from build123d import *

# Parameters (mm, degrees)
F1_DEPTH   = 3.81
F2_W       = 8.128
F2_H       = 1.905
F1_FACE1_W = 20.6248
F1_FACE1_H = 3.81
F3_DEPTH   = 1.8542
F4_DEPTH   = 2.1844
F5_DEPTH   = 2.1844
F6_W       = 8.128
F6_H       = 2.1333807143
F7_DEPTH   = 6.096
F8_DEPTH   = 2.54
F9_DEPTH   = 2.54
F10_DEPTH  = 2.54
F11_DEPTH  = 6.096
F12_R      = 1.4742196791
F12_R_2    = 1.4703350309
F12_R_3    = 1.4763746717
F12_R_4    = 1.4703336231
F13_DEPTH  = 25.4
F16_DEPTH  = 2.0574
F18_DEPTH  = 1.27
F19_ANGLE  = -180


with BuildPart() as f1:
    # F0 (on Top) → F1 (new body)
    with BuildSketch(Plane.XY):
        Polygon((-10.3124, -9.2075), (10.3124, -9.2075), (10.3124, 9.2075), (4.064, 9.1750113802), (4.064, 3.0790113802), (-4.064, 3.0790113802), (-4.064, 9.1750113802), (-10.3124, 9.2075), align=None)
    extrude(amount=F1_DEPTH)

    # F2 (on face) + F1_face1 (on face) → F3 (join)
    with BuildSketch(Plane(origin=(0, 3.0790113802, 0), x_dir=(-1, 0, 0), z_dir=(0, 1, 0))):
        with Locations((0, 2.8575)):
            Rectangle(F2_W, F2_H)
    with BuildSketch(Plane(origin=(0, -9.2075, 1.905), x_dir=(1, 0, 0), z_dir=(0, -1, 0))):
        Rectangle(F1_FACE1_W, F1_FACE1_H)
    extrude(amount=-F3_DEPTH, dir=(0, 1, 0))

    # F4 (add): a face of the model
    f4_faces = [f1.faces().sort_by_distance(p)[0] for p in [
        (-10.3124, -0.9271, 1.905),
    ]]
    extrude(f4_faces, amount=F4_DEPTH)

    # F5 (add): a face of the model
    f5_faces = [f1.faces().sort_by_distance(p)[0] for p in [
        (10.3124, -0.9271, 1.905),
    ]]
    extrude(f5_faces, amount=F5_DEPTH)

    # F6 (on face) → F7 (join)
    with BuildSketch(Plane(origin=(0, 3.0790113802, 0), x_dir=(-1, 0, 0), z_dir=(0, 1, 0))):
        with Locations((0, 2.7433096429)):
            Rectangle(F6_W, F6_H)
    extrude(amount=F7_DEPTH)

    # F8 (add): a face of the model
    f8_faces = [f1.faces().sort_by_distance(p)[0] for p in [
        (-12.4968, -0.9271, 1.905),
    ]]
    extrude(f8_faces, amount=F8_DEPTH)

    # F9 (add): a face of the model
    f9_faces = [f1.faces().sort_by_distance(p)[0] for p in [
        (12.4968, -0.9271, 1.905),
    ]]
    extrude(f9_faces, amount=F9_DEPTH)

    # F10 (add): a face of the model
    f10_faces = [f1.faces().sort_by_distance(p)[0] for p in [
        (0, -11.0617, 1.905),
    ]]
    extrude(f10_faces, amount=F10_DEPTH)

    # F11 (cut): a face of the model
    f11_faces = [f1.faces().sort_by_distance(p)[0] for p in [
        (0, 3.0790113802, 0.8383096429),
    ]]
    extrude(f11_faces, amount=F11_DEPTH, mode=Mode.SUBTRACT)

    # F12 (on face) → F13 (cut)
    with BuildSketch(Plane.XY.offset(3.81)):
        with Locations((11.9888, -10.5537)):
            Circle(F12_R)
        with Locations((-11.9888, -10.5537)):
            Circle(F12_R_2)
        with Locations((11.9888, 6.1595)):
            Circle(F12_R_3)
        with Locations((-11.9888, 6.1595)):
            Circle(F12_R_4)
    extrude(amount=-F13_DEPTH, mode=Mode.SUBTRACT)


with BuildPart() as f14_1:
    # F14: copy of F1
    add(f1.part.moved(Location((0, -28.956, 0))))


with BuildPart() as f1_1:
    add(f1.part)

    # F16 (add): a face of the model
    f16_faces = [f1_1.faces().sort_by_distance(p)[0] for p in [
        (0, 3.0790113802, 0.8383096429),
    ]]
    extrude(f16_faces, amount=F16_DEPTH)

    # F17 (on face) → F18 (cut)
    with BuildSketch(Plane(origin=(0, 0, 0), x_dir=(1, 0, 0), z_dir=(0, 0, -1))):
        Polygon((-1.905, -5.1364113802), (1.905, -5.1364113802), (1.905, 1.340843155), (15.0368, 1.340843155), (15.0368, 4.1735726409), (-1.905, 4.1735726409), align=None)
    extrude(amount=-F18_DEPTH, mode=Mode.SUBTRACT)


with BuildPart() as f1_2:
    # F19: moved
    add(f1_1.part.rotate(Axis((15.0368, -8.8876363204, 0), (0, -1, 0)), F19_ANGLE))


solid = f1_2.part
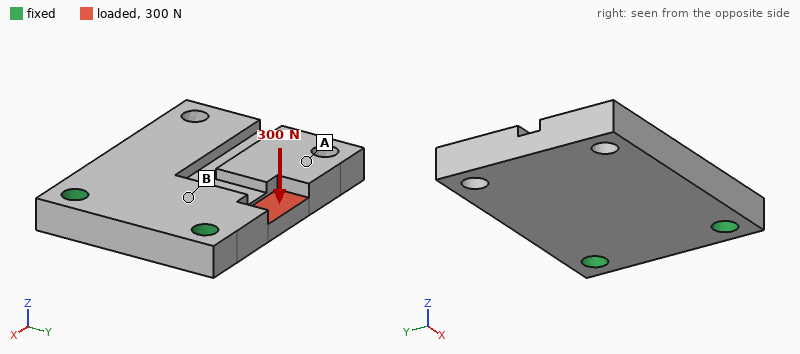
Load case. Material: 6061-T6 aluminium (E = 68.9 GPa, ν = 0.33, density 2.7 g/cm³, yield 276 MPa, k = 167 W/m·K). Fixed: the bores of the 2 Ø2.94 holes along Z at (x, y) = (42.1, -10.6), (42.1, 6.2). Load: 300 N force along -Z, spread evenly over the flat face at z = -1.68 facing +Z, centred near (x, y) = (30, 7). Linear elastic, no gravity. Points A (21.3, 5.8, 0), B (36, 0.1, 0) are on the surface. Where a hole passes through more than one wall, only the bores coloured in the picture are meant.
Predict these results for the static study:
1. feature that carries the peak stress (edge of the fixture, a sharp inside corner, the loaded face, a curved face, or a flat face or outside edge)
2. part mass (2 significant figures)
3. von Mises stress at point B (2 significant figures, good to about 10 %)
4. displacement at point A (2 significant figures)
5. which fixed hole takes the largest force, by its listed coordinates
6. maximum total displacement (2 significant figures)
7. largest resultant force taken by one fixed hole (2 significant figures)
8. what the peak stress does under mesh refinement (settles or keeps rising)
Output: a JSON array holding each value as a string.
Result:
["edge of the fixture", "6.4 g", "39 MPa", "0.081 mm", "(42.1, 6.2)", "0.11 mm", "310 N", "keeps rising"]
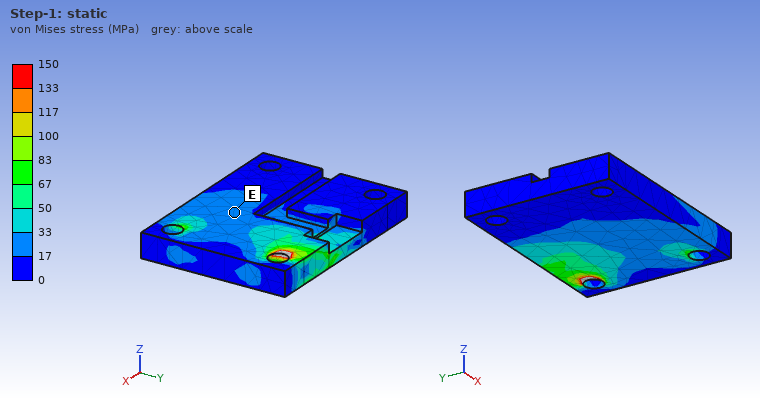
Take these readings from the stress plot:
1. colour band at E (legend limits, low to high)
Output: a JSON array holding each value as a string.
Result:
["17 to 33 MPa"]
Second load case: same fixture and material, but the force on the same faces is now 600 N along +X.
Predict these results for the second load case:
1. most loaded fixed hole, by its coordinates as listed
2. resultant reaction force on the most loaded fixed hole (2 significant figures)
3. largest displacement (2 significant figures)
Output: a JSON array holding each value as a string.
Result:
["(42.1, 6.2)", "630 N", "27 µm"]
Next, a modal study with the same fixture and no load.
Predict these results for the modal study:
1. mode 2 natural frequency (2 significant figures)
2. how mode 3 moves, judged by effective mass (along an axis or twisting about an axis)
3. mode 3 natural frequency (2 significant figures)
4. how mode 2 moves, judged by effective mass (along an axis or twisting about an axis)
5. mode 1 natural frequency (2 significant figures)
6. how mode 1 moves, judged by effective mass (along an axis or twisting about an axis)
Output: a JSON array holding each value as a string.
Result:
["10 kHz", "along Y", "18 kHz", "twisting about X", "4000 Hz", "along Z"]
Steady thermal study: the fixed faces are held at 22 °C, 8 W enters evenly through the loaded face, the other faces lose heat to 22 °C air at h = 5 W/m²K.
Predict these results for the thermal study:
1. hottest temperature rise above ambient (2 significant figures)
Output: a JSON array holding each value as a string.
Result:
["14 K"]
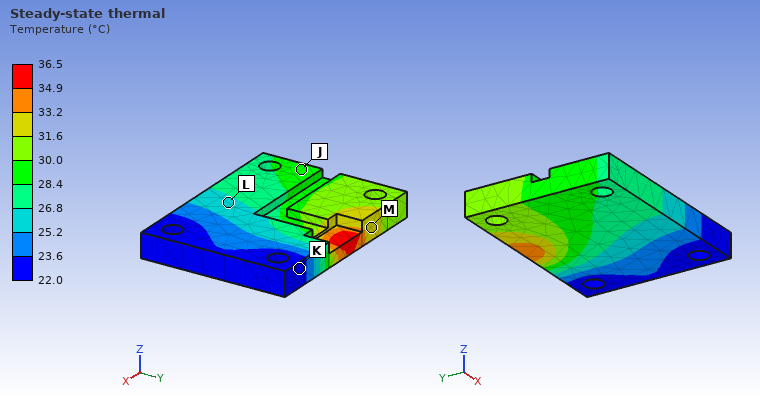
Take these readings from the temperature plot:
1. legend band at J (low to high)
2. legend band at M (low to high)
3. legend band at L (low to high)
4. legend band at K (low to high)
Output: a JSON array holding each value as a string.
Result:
["28.4 to 30.0 °C", "31.6 to 33.2 °C", "25.2 to 26.8 °C", "22.0 to 23.6 °C"]
